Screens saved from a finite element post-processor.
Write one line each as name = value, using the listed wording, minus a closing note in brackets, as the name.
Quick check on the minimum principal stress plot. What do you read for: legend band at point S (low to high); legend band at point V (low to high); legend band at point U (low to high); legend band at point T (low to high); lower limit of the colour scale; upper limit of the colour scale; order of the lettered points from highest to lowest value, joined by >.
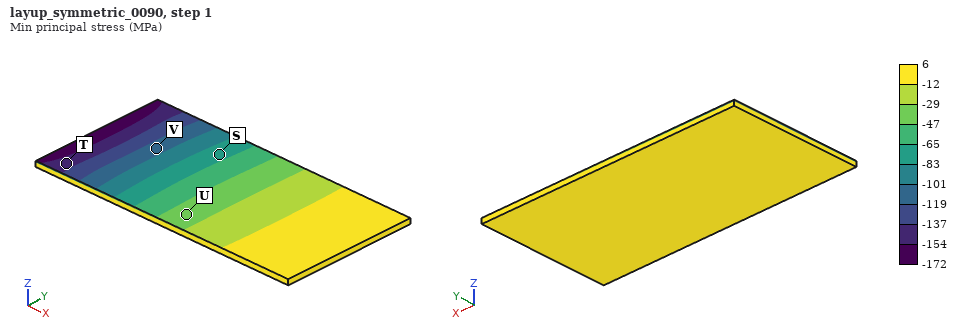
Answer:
legend band at point S = -83 to -65 MPa
legend band at point V = -119 to -101 MPa
legend band at point U = -47 to -29 MPa
legend band at point T = -154 to -137 MPa
lower limit of the colour scale = -172 MPa
upper limit of the colour scale = 6 MPa
order of the lettered points from highest to lowest value, joined by > = U > S > V > T
